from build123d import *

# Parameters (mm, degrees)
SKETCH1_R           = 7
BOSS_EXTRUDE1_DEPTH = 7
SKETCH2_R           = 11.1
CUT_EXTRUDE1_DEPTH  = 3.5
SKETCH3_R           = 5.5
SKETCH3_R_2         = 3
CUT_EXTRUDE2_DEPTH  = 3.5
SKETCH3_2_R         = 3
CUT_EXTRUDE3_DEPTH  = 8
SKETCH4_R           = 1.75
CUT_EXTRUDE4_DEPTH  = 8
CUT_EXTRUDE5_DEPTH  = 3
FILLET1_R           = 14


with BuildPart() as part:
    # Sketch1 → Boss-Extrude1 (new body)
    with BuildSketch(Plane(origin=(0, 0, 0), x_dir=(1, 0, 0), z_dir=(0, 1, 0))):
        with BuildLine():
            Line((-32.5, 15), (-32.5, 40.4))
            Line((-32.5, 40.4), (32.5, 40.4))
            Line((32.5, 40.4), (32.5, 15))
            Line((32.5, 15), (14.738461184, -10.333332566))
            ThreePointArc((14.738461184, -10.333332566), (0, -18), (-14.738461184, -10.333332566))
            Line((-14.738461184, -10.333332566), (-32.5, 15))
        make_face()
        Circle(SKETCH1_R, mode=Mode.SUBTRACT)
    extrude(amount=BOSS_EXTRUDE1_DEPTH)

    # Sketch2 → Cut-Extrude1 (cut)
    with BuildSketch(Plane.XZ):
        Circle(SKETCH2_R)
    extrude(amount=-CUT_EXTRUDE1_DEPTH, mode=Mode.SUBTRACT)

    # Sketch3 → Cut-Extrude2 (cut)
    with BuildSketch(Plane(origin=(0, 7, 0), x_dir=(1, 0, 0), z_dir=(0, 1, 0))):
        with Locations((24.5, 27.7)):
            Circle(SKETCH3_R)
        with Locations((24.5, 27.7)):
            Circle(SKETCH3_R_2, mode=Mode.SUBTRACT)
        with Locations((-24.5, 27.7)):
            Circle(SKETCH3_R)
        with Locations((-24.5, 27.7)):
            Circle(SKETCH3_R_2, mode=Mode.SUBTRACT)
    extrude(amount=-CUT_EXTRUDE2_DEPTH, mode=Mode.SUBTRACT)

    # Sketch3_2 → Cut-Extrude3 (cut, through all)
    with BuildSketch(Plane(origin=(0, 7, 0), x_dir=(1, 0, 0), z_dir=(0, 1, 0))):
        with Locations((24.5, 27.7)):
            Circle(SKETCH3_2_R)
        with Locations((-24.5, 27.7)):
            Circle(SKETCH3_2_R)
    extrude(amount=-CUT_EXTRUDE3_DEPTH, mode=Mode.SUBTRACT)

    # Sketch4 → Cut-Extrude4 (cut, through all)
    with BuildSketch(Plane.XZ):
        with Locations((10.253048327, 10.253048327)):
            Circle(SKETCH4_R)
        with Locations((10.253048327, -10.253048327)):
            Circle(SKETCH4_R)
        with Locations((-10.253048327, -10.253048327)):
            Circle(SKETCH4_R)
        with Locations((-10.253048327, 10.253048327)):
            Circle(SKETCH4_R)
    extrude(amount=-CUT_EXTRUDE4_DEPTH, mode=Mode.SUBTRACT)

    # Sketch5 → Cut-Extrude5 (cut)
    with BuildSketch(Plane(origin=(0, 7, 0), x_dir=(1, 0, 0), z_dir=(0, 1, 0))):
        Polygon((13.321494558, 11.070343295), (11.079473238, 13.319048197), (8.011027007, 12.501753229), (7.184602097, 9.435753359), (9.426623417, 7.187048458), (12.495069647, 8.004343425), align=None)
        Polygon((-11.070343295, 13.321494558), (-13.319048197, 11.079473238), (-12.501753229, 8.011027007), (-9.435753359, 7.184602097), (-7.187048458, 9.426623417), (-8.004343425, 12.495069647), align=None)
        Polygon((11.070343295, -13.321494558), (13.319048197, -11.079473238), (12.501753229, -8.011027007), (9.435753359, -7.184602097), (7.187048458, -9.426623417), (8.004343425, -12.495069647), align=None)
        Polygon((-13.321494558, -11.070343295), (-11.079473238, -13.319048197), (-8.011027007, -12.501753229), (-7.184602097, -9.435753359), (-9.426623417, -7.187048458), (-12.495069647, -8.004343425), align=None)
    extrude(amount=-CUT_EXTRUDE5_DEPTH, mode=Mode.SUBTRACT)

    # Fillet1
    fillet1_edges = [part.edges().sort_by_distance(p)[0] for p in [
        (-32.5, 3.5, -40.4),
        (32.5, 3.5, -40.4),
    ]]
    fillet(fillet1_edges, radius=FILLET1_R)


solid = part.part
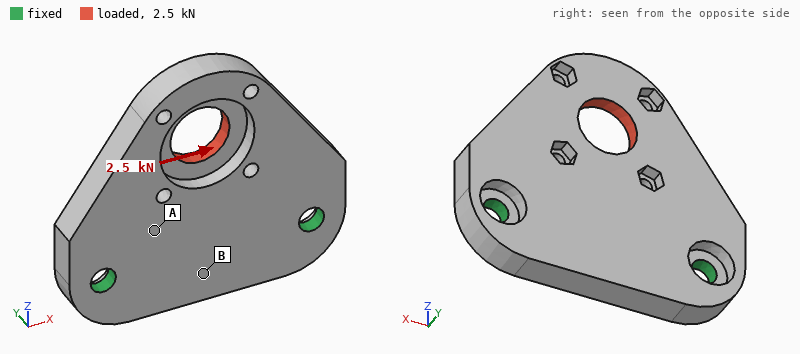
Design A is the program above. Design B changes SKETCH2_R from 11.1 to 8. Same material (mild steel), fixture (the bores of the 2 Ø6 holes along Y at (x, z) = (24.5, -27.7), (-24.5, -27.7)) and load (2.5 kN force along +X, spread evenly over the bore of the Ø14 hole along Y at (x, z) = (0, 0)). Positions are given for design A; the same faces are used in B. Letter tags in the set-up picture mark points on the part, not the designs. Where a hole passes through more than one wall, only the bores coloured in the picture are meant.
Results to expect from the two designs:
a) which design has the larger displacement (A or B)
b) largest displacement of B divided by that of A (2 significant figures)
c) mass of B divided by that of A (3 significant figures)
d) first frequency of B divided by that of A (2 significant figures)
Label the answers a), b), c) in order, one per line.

a) A
b) 0.90
c) 1.04
d) 0.97
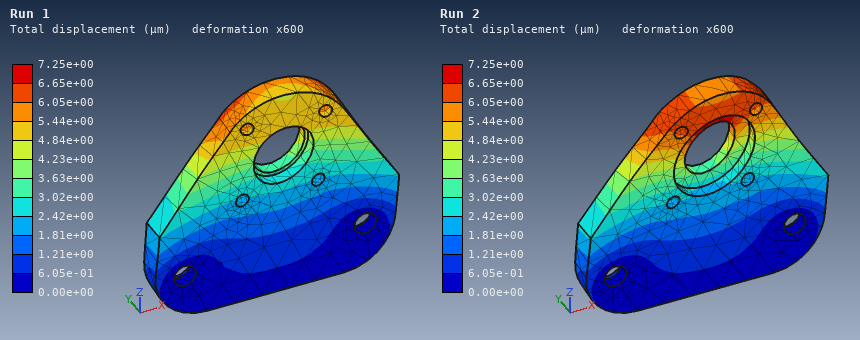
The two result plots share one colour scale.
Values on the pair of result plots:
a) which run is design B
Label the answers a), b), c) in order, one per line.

a) Run 1
